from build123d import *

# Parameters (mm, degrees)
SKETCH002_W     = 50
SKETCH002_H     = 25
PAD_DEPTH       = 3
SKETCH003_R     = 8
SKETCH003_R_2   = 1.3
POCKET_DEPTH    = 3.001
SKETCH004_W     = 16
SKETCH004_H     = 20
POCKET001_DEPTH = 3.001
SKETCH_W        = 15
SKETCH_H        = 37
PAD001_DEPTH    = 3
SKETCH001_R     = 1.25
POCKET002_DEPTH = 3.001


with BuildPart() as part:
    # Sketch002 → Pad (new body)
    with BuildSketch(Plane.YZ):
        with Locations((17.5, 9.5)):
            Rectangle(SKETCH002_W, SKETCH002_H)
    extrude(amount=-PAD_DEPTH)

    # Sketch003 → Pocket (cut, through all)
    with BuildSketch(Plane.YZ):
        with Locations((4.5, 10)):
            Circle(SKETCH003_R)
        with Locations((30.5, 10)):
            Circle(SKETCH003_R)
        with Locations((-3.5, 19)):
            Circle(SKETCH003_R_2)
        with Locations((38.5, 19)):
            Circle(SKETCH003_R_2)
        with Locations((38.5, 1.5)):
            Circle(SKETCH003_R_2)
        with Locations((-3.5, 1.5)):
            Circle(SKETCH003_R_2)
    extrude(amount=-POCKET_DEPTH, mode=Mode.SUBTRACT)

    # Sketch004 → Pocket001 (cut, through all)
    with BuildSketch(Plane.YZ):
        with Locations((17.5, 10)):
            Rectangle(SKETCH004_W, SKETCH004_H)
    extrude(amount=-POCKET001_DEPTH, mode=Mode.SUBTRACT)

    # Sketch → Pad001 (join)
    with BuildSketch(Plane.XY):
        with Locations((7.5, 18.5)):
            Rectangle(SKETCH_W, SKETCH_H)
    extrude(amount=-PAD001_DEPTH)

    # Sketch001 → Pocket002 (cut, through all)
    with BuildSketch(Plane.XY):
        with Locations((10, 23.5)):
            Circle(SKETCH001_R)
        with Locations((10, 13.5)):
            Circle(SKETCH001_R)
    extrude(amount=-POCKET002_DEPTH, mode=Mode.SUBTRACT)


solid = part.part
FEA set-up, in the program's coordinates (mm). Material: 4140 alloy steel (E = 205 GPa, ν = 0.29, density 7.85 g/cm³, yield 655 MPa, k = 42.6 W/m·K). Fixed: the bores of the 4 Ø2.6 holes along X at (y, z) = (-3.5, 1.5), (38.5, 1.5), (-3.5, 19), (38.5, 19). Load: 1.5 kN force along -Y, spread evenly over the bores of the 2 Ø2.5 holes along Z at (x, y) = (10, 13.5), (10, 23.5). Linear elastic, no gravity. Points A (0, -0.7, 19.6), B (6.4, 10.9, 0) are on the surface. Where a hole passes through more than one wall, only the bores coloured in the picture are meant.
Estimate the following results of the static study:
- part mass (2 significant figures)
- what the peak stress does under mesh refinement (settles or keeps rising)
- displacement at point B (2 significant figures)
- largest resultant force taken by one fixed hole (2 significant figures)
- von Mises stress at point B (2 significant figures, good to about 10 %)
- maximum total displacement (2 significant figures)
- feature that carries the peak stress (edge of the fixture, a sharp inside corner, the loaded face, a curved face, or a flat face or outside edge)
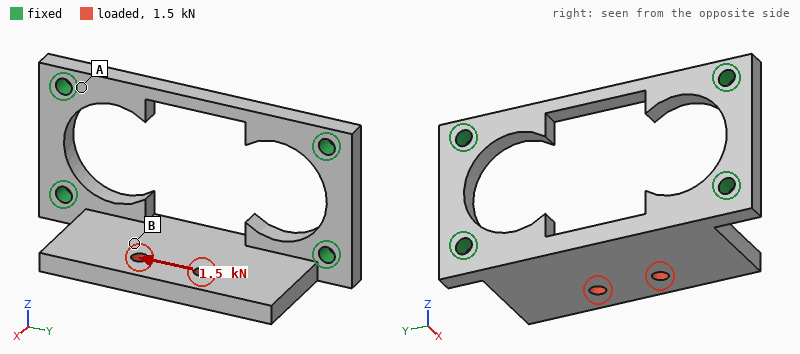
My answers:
26 g
keeps rising
6.5 µm
910 N
37 MPa
12 µm
edge of the fixture
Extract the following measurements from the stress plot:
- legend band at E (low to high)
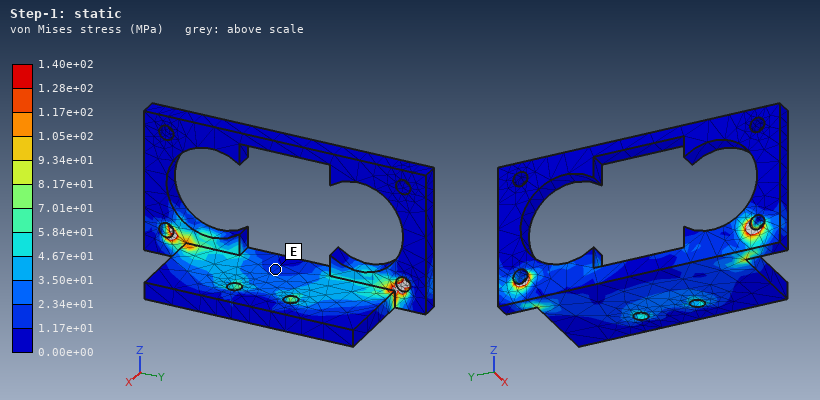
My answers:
1.17e+01 to 2.34e+01 MPa
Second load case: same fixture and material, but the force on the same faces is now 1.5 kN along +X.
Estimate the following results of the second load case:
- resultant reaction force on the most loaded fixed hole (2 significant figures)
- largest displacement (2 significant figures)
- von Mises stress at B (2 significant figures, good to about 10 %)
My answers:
910 N
33 µm
40 MPa
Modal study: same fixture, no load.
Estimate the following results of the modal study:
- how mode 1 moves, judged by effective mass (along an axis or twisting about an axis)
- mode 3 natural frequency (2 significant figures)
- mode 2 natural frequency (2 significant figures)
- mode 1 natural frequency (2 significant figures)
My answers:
along Z
11 kHz
9900 Hz
4100 Hz
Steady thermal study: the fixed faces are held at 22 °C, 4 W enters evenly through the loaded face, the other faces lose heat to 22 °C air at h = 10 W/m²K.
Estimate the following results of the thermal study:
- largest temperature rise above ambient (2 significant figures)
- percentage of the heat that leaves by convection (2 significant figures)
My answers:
30 K
8.9 %
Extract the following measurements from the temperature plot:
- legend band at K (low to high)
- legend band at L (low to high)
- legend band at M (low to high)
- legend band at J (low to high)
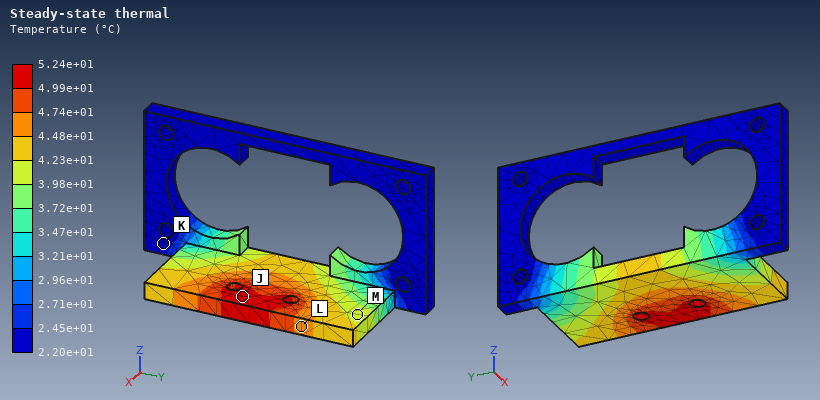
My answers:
2.20e+01 to 2.45e+01 °C
4.48e+01 to 4.74e+01 °C
3.98e+01 to 4.23e+01 °C
4.99e+01 to 5.24e+01 °C
